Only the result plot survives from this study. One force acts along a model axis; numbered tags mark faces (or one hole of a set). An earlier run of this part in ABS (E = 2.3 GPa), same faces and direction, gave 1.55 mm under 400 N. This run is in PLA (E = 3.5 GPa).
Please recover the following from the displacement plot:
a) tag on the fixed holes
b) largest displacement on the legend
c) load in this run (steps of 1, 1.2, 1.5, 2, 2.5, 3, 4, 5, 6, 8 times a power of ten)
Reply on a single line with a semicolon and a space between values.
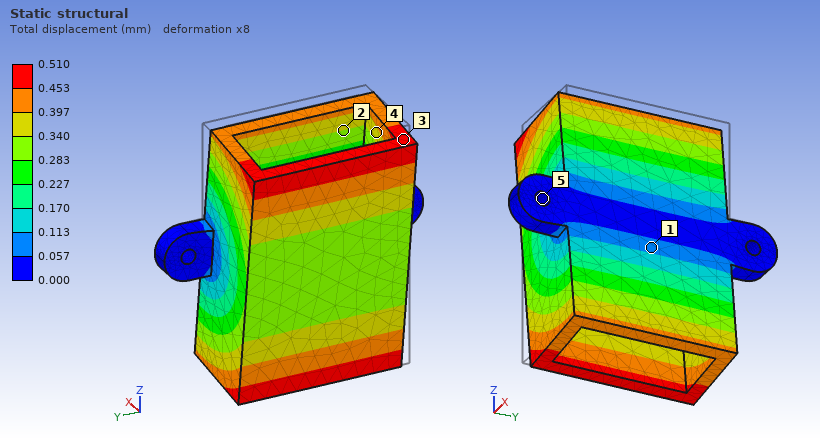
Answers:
5; 0.510 mm; 200 N
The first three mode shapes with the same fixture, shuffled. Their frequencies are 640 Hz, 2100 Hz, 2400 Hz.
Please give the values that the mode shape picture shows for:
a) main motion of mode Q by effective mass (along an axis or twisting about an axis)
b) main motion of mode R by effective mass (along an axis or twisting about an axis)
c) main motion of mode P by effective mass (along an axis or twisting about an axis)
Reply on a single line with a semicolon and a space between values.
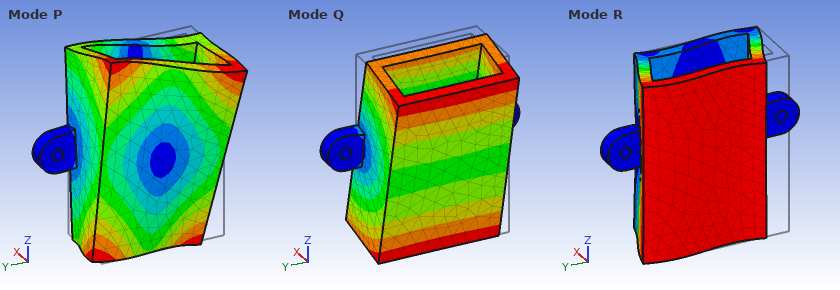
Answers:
along Z; along Y; twisting about X
